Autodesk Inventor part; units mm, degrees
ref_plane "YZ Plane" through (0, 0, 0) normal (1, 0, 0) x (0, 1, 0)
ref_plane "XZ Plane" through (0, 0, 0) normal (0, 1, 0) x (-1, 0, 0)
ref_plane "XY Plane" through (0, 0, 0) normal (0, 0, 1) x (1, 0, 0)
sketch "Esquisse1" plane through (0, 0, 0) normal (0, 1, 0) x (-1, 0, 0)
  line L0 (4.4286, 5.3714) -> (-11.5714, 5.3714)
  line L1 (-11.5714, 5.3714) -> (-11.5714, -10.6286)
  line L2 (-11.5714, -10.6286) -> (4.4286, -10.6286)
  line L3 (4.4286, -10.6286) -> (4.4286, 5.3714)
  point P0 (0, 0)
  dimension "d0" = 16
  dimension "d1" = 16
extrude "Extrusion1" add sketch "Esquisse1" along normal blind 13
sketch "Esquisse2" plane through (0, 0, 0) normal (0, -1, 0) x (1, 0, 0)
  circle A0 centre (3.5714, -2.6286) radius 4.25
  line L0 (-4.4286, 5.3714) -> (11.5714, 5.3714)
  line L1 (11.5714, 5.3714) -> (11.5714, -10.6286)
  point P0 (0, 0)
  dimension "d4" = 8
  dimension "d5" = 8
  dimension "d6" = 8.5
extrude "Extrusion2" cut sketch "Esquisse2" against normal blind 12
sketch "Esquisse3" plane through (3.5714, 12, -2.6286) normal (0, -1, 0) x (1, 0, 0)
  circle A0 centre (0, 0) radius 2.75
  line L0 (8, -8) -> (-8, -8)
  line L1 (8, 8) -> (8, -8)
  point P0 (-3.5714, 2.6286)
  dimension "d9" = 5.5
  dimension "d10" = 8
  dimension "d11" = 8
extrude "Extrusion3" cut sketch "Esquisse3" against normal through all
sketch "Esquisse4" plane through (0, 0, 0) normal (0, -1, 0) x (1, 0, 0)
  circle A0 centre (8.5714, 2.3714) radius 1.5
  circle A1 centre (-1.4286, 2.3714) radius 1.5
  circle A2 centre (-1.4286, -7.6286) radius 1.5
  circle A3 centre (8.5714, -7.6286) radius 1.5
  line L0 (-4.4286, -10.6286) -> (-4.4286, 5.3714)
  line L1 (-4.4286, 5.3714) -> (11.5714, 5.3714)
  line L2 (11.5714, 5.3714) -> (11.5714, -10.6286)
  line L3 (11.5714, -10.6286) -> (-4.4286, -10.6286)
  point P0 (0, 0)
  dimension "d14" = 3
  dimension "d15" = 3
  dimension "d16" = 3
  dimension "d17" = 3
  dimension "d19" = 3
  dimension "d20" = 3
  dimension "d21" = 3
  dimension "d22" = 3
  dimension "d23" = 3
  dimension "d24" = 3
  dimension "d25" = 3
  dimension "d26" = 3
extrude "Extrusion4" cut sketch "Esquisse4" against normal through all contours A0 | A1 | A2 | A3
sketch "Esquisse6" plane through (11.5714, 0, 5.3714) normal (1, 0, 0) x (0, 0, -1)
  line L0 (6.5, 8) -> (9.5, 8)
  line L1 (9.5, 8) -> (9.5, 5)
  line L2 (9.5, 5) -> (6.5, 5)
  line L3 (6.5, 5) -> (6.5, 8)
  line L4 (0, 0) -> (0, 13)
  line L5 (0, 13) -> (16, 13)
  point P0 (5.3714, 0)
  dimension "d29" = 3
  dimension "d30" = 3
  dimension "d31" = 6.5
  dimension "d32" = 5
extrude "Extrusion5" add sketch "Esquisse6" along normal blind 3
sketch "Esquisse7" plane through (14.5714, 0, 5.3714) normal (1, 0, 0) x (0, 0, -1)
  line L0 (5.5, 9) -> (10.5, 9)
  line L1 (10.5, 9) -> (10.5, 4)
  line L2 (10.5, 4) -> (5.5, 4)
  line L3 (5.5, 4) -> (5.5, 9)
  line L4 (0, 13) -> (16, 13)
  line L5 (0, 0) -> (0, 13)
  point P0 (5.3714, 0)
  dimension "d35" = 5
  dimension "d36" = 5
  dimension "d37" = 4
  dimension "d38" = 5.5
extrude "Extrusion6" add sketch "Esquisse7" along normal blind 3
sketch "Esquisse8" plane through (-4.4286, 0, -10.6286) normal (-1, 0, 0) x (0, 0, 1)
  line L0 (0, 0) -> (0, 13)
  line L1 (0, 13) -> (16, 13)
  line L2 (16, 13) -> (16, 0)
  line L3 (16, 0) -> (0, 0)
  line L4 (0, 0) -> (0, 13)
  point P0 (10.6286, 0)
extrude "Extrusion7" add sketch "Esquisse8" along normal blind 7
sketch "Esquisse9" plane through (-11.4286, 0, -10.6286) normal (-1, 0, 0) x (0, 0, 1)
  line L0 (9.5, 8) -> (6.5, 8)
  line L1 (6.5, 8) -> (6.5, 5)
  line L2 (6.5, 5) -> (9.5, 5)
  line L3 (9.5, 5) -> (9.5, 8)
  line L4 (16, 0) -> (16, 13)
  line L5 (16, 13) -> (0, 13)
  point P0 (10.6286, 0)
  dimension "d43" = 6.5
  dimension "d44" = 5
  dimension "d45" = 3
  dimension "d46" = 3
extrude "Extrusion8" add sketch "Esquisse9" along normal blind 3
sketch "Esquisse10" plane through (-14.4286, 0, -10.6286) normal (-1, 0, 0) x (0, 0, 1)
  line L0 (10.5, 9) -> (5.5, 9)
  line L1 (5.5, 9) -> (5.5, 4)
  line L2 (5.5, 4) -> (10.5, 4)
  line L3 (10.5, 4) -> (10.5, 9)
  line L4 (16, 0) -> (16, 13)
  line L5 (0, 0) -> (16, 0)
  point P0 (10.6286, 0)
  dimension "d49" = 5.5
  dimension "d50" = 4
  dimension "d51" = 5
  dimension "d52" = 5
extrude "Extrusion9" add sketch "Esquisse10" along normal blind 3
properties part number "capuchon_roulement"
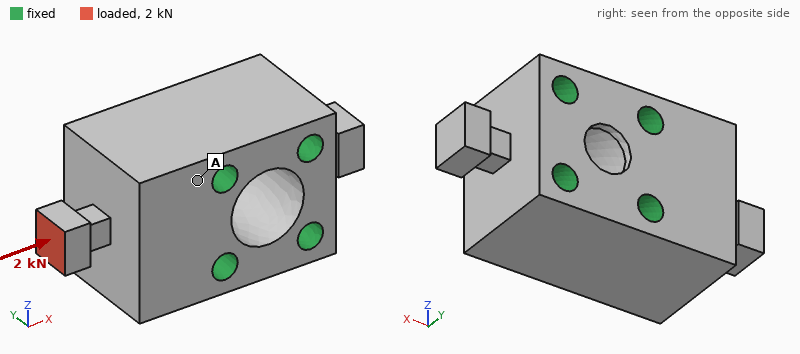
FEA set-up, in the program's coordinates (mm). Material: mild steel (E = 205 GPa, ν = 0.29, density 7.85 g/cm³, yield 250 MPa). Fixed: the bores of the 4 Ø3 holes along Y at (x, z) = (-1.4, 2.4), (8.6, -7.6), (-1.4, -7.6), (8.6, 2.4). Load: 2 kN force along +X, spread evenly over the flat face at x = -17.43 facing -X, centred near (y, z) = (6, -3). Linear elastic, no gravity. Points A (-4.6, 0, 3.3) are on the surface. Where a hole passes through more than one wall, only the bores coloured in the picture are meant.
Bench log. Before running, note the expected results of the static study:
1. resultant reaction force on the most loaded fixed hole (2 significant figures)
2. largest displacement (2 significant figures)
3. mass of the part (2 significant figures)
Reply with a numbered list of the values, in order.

1. 1.1 kN
2. 7.5 µm
3. 31 g
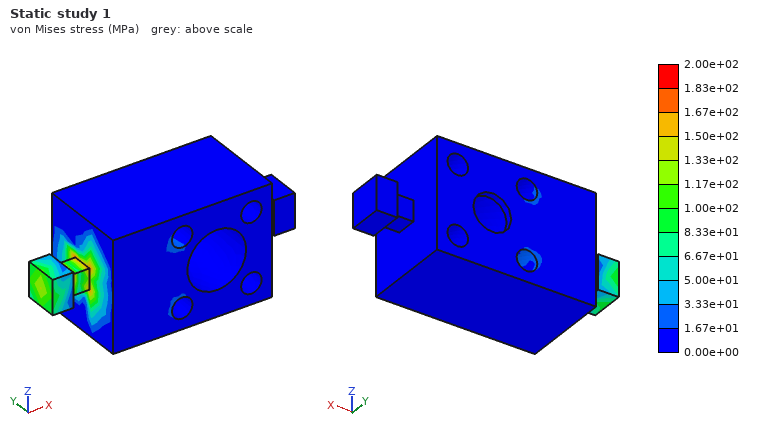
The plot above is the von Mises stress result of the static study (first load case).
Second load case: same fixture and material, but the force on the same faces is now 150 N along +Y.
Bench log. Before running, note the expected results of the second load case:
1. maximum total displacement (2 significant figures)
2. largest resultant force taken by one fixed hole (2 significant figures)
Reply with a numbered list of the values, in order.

1. 13 µm
2. 77 N
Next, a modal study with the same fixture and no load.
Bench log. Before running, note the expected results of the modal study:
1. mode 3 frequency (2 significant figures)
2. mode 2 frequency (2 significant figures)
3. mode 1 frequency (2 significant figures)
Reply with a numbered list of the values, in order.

1. 30 kHz
2. 30 kHz
3. 30 kHz
